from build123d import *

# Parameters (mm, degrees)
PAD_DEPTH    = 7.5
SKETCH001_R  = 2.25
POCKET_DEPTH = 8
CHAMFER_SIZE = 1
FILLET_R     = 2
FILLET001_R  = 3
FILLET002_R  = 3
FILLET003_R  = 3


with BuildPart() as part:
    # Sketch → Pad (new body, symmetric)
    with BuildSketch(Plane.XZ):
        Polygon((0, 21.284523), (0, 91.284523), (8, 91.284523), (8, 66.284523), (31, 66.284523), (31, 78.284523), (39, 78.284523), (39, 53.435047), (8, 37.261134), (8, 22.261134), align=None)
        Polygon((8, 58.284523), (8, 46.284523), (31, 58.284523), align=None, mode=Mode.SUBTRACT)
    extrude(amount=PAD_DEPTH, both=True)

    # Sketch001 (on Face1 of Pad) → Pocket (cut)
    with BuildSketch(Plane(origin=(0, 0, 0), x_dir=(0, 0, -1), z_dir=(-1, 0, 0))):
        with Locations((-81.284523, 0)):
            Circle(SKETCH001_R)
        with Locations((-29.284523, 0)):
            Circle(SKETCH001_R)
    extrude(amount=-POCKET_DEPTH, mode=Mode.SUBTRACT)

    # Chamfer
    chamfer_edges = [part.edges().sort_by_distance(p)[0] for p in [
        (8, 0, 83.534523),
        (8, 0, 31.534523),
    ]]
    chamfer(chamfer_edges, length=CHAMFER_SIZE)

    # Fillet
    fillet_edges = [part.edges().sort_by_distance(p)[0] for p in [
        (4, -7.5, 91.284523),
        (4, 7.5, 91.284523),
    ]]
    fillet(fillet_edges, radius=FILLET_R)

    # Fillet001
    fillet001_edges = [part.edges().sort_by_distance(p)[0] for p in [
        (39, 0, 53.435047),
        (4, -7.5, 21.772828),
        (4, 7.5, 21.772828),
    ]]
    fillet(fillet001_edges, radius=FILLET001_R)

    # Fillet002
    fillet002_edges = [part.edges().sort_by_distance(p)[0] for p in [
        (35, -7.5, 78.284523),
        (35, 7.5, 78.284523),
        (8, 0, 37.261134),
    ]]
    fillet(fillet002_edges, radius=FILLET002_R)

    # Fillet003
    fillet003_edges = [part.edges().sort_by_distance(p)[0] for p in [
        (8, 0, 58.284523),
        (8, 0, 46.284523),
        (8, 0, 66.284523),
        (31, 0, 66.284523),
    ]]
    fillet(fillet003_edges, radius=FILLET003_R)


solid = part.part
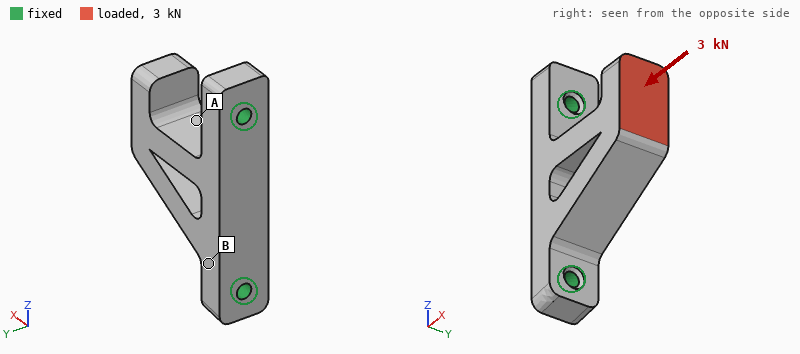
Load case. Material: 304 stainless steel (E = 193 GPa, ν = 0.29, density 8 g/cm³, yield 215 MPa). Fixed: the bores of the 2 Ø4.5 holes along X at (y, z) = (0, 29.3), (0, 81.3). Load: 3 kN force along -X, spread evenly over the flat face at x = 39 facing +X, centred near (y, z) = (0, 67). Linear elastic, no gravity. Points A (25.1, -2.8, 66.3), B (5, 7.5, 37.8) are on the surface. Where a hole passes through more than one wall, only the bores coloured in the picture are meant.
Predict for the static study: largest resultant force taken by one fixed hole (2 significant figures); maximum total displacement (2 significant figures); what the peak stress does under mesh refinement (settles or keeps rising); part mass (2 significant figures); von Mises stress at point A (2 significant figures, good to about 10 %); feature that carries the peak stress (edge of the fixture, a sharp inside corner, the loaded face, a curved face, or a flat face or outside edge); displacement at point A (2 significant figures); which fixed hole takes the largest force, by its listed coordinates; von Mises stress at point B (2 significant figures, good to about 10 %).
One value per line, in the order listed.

2.4 kN
45 µm
keeps rising
140 g
64 MPa
edge of the fixture
20 µm
(0, 81.3)
15 MPa
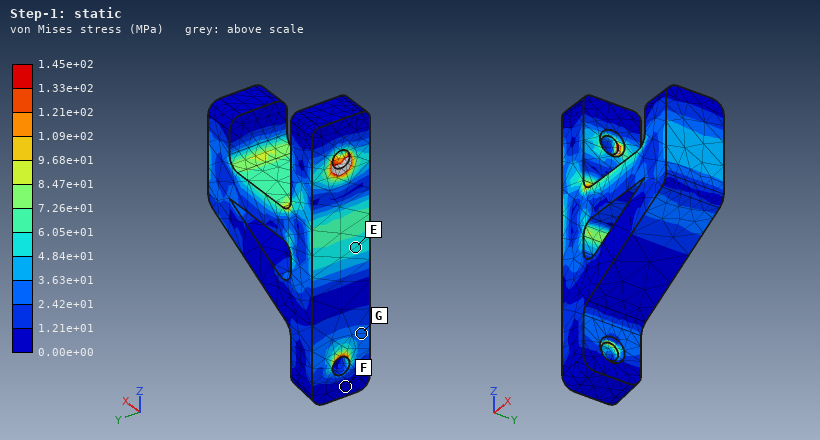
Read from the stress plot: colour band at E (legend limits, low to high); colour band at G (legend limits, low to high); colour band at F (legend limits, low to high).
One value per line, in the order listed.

4.84e+01 to 6.05e+01 MPa
2.42e+01 to 3.63e+01 MPa
0.00e+00 to 1.21e+01 MPa
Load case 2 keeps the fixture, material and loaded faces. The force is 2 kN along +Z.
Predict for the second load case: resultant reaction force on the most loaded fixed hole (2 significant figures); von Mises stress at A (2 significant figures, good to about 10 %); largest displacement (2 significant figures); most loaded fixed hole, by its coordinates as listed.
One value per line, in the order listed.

2.1 kN
23 MPa
36 µm
(0, 29.3)
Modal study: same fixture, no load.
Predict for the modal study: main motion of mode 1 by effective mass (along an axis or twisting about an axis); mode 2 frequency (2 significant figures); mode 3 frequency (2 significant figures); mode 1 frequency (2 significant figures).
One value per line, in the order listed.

along Y
6700 Hz
11 kHz
3100 Hz
